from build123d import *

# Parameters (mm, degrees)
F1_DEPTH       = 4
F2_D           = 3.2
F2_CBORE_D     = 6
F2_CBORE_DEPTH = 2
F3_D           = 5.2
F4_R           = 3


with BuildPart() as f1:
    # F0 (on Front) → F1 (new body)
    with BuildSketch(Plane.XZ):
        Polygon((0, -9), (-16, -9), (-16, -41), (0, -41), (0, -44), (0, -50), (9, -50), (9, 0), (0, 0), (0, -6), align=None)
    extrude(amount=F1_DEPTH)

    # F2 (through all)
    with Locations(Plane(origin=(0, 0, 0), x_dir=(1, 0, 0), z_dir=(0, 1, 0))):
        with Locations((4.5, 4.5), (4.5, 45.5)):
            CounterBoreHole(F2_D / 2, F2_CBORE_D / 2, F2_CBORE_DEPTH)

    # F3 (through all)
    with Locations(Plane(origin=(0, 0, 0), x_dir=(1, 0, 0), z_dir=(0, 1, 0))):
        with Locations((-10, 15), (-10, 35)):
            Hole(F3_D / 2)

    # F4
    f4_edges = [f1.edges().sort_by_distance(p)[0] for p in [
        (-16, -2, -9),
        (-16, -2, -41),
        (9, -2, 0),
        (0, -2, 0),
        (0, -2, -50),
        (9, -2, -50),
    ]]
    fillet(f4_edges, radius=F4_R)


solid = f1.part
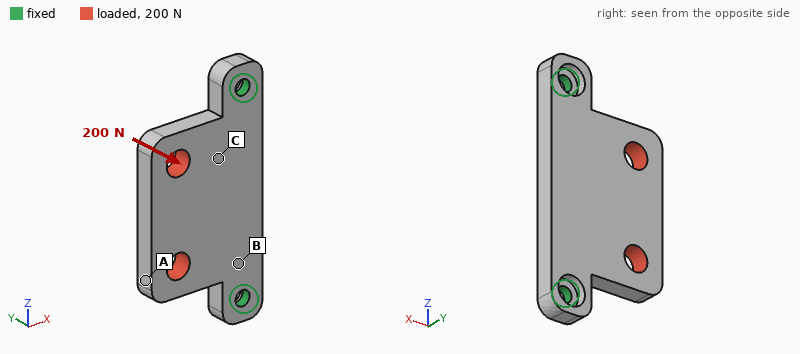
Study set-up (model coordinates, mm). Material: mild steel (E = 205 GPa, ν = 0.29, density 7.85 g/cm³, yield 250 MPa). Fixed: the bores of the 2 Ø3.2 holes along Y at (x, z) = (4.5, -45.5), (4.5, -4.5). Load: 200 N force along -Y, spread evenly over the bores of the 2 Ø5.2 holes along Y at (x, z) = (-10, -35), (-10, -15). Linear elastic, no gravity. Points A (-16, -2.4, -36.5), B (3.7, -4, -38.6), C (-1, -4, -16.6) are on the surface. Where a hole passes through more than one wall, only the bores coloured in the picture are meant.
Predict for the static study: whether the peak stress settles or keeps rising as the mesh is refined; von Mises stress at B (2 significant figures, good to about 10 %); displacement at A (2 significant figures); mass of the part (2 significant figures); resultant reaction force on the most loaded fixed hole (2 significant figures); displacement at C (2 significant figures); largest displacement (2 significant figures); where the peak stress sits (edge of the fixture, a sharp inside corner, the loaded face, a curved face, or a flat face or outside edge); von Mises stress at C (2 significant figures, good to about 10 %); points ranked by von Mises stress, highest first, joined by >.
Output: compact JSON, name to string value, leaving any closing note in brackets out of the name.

{"whether the peak stress settles or keeps rising as the mesh is refined": "keeps rising", "von Mises stress at B": "48 MPa", "displacement at A": "42 µm", "mass of the part": "27 g", "resultant reaction force on the most loaded fixed hole": "150 N", "displacement at C": "12 µm", "largest displacement": "44 µm", "where the peak stress sits": "edge of the fixture", "von Mises stress at C": "23 MPa", "points ranked by von Mises stress, highest first, joined by >": "B > C > A"}
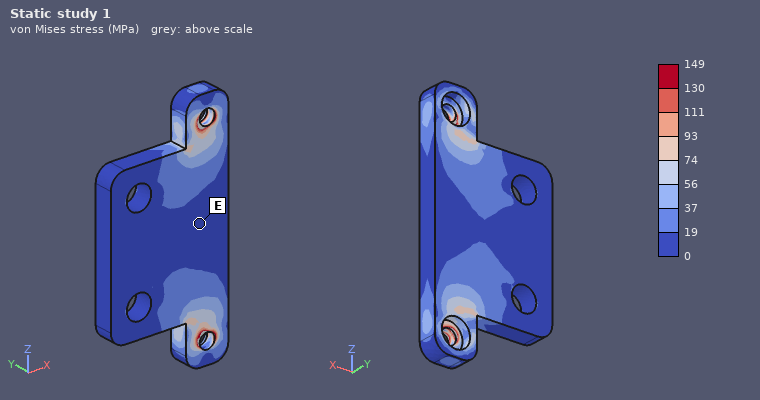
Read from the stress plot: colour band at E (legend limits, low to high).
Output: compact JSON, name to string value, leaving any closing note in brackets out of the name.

{"colour band at E": "0 to 19 MPa"}
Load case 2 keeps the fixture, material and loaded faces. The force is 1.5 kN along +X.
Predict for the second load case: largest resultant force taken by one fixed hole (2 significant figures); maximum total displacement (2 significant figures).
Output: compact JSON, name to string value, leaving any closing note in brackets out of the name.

{"largest resultant force taken by one fixed hole": "800 N", "maximum total displacement": "14 µm"}
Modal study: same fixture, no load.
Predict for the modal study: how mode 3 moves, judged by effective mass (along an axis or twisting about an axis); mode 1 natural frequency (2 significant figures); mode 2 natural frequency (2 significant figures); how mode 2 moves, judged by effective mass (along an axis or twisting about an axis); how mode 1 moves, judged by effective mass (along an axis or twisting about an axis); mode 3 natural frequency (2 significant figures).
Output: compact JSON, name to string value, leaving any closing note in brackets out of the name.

{"how mode 3 moves, judged by effective mass": "twisting about X", "mode 1 natural frequency": "3600 Hz", "mode 2 natural frequency": "11 kHz", "how mode 2 moves, judged by effective mass": "along Y", "how mode 1 moves, judged by effective mass": "along Y", "mode 3 natural frequency": "11 kHz"}
